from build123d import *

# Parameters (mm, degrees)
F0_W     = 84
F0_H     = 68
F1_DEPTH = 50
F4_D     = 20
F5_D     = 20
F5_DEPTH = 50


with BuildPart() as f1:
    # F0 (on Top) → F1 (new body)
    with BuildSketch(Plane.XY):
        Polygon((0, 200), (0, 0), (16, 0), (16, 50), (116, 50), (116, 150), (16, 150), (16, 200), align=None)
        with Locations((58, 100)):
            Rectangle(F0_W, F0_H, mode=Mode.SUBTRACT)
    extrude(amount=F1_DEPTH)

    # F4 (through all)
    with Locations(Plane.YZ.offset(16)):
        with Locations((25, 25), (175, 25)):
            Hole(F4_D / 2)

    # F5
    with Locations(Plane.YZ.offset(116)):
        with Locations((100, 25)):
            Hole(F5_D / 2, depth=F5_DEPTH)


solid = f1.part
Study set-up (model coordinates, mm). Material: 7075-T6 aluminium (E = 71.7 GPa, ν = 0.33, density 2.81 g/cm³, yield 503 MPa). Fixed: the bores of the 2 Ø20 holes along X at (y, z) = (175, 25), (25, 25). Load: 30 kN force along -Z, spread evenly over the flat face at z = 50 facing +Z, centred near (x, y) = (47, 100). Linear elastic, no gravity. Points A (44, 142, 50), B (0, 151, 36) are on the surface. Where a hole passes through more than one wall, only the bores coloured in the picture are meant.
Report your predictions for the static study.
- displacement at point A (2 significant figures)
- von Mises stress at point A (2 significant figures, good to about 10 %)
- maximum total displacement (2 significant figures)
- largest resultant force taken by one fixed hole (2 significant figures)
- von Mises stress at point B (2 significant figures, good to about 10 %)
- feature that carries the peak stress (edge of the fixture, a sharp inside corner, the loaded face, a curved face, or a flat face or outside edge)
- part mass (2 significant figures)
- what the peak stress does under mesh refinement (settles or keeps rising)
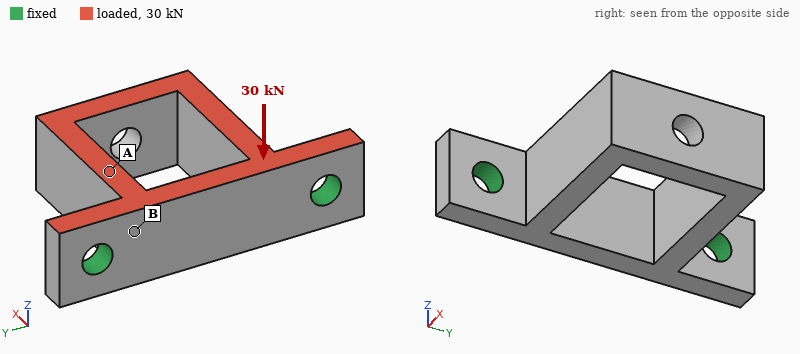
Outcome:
0.36 mm
47 MPa
0.93 mm
15 kN
100 MPa
edge of the fixture
1.0 kg
keeps rising
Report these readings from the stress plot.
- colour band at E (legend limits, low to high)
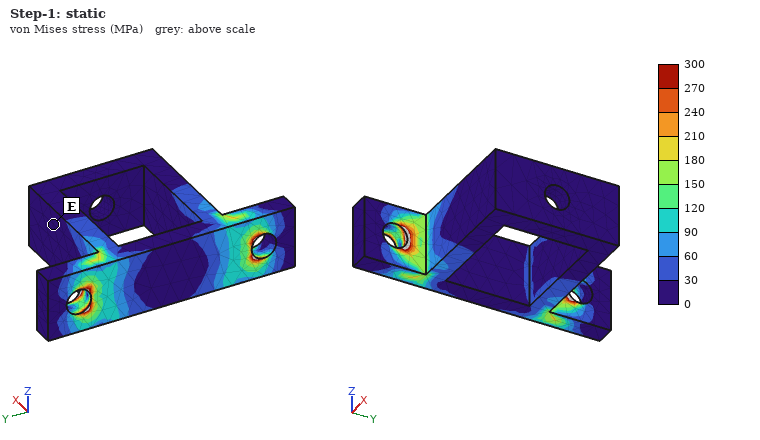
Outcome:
0 to 30 MPa
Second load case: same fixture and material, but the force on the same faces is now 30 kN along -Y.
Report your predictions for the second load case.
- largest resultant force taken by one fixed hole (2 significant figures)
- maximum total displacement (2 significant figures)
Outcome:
18 kN
0.63 mm
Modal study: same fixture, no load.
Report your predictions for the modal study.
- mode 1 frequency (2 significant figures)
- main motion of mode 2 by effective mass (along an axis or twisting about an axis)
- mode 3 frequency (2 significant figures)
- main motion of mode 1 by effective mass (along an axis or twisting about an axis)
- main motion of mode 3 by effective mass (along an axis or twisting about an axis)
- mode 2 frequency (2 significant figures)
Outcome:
1000 Hz
along Y
2200 Hz
along Z
twisting about X
1300 Hz
